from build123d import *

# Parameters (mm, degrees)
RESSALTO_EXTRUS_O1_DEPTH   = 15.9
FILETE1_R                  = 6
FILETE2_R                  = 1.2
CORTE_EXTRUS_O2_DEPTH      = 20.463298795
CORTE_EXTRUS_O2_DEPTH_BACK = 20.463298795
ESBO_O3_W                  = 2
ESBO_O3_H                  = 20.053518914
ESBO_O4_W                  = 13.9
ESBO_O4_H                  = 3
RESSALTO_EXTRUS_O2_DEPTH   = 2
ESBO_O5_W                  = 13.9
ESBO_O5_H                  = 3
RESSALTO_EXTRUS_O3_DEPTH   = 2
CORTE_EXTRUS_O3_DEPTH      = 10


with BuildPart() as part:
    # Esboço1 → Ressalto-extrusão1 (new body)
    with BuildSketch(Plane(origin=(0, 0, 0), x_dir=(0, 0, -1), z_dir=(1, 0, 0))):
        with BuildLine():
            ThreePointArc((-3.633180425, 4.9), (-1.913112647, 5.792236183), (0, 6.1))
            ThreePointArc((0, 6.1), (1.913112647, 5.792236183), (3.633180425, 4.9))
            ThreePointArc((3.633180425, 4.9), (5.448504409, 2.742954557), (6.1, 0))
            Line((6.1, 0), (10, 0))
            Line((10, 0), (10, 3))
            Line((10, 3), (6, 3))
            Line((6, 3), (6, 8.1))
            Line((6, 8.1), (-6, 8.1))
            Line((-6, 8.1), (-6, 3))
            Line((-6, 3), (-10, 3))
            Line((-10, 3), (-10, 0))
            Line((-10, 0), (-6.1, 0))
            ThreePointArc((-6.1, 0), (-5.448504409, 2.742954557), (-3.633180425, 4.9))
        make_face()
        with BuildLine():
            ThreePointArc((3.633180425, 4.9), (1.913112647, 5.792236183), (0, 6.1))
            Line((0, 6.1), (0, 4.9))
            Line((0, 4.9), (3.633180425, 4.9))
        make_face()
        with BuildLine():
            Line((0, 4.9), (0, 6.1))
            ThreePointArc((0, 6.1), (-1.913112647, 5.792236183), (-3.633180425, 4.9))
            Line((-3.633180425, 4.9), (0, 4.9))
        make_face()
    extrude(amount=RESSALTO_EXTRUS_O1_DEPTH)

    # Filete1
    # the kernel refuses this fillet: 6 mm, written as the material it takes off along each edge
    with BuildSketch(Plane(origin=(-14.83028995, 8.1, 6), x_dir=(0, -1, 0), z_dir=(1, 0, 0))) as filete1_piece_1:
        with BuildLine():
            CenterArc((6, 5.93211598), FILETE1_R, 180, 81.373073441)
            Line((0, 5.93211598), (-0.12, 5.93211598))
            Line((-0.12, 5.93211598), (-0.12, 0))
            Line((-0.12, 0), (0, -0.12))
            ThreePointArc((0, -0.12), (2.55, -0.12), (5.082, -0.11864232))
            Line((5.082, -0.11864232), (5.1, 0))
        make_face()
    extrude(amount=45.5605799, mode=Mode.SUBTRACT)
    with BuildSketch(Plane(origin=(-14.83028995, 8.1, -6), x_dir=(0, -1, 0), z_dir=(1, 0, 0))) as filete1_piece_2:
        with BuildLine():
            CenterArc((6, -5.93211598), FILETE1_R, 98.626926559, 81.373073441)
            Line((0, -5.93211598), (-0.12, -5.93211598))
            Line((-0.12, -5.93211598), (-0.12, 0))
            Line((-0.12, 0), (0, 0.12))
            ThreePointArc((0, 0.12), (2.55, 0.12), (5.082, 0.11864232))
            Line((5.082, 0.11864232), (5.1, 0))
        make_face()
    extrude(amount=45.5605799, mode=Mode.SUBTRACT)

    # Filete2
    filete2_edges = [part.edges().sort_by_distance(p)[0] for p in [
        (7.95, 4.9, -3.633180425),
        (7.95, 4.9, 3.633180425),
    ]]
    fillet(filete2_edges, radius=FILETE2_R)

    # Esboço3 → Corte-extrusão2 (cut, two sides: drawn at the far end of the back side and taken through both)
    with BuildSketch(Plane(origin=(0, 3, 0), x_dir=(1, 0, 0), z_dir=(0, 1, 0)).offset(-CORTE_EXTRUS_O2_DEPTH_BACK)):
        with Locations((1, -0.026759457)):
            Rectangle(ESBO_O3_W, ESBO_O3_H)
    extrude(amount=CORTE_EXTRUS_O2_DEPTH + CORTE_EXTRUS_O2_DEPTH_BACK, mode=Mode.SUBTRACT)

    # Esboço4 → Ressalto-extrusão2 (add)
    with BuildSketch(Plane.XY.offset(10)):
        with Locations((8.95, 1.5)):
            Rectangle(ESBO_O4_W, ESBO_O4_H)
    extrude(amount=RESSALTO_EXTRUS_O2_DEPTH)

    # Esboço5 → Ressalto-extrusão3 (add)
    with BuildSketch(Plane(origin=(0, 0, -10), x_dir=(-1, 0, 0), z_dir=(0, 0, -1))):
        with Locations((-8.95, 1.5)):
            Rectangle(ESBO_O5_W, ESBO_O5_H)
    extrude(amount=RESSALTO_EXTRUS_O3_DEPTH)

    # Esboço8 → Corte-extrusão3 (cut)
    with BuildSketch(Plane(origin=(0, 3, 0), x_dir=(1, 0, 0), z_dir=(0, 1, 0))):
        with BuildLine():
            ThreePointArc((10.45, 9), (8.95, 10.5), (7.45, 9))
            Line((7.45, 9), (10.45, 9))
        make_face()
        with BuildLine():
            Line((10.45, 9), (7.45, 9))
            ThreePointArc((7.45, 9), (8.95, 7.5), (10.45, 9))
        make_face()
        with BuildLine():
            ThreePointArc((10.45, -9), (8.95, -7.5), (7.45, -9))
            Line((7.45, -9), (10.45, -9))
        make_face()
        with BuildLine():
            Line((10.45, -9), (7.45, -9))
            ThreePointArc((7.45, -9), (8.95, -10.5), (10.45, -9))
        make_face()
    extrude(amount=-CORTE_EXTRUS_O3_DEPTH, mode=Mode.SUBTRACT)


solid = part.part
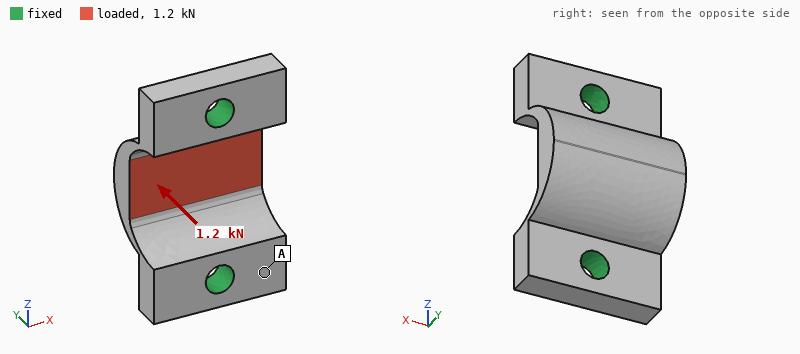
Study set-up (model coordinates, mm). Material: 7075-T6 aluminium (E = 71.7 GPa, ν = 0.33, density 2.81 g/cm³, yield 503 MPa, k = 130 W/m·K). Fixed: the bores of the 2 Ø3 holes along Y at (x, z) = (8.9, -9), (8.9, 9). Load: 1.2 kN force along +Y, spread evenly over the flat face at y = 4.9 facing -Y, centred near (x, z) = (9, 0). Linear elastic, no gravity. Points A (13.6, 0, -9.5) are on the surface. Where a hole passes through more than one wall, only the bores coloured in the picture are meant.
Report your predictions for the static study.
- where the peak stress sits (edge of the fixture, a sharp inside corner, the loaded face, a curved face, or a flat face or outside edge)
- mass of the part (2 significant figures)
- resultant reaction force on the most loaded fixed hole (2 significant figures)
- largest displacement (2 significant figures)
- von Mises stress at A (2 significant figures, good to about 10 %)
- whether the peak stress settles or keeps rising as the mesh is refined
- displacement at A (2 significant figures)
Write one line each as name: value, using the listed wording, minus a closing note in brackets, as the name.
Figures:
where the peak stress sits: edge of the fixture
mass of the part: 2.5 g
resultant reaction force on the most loaded fixed hole: 740 N
largest displacement: 15 µm
von Mises stress at A: 17 MPa
whether the peak stress settles or keeps rising as the mesh is refined: keeps rising
displacement at A: 3.5 µm
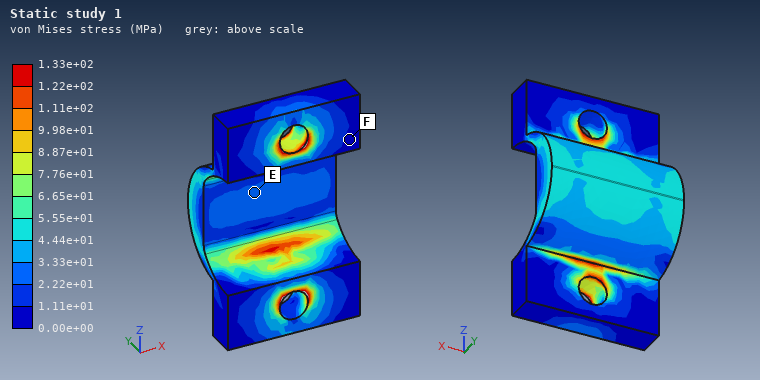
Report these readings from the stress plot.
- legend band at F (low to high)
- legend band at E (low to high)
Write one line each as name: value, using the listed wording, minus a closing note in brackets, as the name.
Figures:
legend band at F: 0.00e+00 to 1.11e+01 MPa
legend band at E: 2.22e+01 to 3.33e+01 MPa
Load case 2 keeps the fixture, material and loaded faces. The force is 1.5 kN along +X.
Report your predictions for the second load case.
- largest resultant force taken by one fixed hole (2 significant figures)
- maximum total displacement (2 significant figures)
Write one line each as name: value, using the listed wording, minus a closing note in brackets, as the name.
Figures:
largest resultant force taken by one fixed hole: 750 N
maximum total displacement: 44 µm
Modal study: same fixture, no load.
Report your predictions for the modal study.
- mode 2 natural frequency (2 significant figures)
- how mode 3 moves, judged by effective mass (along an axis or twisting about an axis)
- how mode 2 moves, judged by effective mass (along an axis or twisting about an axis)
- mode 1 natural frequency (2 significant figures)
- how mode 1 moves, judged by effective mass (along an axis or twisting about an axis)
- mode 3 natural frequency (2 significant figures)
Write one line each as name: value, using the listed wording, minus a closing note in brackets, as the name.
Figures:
mode 2 natural frequency: 37 kHz
how mode 3 moves, judged by effective mass: along Y
how mode 2 moves, judged by effective mass: along Z
mode 1 natural frequency: 25 kHz
how mode 1 moves, judged by effective mass: along X
mode 3 natural frequency: 48 kHz
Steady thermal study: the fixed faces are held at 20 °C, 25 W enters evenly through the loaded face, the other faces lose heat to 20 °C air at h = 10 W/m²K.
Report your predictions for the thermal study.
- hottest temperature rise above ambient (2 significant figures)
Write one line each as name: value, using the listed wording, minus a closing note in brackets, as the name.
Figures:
hottest temperature rise above ambient: 46 K
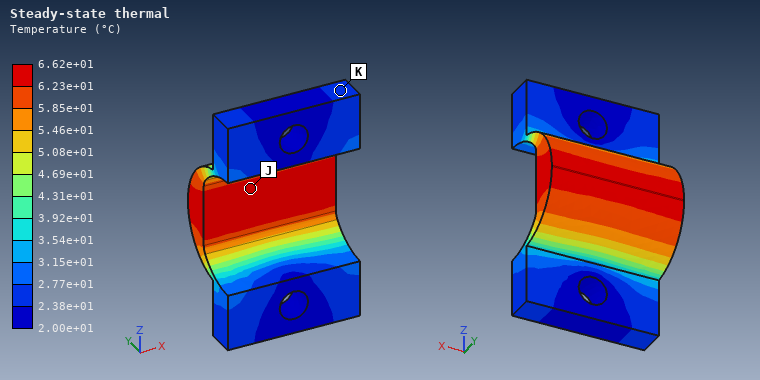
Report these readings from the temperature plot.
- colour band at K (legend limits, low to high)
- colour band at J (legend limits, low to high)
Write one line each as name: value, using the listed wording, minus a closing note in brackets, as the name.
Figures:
colour band at K: 2.38e+01 to 2.77e+01 °C
colour band at J: 6.23e+01 to 6.62e+01 °C
